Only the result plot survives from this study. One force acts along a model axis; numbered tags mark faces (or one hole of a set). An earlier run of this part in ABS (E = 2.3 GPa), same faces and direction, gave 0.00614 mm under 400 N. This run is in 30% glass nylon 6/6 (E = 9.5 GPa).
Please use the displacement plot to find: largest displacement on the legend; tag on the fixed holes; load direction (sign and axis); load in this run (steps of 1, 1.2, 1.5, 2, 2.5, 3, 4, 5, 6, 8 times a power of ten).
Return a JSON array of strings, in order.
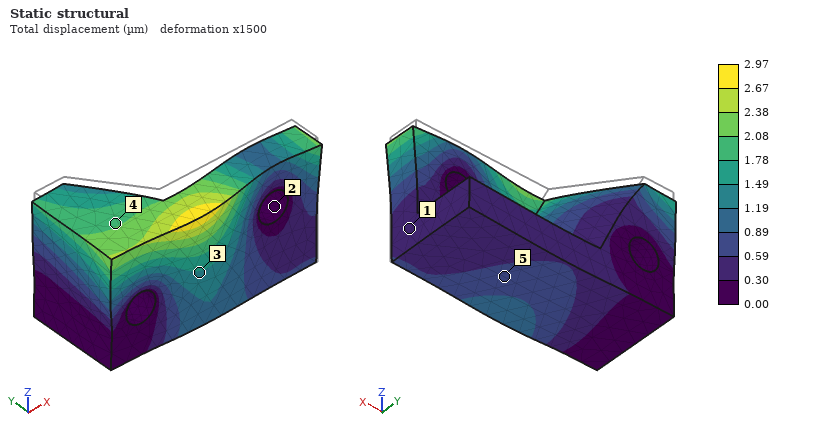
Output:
["2.97 µm", "2", "-Z", "800 N"]
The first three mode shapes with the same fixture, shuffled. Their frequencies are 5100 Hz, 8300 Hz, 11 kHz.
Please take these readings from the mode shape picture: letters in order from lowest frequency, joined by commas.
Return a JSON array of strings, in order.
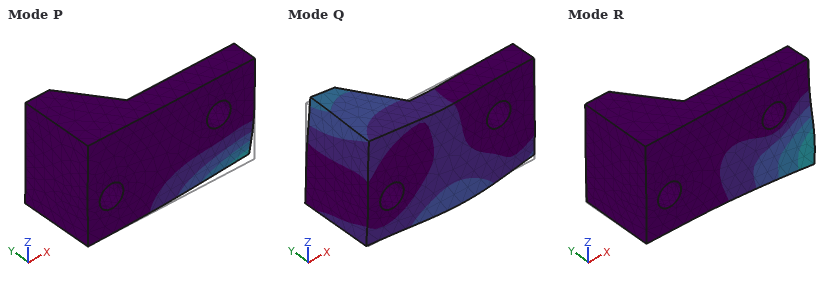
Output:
["P, R, Q"]
